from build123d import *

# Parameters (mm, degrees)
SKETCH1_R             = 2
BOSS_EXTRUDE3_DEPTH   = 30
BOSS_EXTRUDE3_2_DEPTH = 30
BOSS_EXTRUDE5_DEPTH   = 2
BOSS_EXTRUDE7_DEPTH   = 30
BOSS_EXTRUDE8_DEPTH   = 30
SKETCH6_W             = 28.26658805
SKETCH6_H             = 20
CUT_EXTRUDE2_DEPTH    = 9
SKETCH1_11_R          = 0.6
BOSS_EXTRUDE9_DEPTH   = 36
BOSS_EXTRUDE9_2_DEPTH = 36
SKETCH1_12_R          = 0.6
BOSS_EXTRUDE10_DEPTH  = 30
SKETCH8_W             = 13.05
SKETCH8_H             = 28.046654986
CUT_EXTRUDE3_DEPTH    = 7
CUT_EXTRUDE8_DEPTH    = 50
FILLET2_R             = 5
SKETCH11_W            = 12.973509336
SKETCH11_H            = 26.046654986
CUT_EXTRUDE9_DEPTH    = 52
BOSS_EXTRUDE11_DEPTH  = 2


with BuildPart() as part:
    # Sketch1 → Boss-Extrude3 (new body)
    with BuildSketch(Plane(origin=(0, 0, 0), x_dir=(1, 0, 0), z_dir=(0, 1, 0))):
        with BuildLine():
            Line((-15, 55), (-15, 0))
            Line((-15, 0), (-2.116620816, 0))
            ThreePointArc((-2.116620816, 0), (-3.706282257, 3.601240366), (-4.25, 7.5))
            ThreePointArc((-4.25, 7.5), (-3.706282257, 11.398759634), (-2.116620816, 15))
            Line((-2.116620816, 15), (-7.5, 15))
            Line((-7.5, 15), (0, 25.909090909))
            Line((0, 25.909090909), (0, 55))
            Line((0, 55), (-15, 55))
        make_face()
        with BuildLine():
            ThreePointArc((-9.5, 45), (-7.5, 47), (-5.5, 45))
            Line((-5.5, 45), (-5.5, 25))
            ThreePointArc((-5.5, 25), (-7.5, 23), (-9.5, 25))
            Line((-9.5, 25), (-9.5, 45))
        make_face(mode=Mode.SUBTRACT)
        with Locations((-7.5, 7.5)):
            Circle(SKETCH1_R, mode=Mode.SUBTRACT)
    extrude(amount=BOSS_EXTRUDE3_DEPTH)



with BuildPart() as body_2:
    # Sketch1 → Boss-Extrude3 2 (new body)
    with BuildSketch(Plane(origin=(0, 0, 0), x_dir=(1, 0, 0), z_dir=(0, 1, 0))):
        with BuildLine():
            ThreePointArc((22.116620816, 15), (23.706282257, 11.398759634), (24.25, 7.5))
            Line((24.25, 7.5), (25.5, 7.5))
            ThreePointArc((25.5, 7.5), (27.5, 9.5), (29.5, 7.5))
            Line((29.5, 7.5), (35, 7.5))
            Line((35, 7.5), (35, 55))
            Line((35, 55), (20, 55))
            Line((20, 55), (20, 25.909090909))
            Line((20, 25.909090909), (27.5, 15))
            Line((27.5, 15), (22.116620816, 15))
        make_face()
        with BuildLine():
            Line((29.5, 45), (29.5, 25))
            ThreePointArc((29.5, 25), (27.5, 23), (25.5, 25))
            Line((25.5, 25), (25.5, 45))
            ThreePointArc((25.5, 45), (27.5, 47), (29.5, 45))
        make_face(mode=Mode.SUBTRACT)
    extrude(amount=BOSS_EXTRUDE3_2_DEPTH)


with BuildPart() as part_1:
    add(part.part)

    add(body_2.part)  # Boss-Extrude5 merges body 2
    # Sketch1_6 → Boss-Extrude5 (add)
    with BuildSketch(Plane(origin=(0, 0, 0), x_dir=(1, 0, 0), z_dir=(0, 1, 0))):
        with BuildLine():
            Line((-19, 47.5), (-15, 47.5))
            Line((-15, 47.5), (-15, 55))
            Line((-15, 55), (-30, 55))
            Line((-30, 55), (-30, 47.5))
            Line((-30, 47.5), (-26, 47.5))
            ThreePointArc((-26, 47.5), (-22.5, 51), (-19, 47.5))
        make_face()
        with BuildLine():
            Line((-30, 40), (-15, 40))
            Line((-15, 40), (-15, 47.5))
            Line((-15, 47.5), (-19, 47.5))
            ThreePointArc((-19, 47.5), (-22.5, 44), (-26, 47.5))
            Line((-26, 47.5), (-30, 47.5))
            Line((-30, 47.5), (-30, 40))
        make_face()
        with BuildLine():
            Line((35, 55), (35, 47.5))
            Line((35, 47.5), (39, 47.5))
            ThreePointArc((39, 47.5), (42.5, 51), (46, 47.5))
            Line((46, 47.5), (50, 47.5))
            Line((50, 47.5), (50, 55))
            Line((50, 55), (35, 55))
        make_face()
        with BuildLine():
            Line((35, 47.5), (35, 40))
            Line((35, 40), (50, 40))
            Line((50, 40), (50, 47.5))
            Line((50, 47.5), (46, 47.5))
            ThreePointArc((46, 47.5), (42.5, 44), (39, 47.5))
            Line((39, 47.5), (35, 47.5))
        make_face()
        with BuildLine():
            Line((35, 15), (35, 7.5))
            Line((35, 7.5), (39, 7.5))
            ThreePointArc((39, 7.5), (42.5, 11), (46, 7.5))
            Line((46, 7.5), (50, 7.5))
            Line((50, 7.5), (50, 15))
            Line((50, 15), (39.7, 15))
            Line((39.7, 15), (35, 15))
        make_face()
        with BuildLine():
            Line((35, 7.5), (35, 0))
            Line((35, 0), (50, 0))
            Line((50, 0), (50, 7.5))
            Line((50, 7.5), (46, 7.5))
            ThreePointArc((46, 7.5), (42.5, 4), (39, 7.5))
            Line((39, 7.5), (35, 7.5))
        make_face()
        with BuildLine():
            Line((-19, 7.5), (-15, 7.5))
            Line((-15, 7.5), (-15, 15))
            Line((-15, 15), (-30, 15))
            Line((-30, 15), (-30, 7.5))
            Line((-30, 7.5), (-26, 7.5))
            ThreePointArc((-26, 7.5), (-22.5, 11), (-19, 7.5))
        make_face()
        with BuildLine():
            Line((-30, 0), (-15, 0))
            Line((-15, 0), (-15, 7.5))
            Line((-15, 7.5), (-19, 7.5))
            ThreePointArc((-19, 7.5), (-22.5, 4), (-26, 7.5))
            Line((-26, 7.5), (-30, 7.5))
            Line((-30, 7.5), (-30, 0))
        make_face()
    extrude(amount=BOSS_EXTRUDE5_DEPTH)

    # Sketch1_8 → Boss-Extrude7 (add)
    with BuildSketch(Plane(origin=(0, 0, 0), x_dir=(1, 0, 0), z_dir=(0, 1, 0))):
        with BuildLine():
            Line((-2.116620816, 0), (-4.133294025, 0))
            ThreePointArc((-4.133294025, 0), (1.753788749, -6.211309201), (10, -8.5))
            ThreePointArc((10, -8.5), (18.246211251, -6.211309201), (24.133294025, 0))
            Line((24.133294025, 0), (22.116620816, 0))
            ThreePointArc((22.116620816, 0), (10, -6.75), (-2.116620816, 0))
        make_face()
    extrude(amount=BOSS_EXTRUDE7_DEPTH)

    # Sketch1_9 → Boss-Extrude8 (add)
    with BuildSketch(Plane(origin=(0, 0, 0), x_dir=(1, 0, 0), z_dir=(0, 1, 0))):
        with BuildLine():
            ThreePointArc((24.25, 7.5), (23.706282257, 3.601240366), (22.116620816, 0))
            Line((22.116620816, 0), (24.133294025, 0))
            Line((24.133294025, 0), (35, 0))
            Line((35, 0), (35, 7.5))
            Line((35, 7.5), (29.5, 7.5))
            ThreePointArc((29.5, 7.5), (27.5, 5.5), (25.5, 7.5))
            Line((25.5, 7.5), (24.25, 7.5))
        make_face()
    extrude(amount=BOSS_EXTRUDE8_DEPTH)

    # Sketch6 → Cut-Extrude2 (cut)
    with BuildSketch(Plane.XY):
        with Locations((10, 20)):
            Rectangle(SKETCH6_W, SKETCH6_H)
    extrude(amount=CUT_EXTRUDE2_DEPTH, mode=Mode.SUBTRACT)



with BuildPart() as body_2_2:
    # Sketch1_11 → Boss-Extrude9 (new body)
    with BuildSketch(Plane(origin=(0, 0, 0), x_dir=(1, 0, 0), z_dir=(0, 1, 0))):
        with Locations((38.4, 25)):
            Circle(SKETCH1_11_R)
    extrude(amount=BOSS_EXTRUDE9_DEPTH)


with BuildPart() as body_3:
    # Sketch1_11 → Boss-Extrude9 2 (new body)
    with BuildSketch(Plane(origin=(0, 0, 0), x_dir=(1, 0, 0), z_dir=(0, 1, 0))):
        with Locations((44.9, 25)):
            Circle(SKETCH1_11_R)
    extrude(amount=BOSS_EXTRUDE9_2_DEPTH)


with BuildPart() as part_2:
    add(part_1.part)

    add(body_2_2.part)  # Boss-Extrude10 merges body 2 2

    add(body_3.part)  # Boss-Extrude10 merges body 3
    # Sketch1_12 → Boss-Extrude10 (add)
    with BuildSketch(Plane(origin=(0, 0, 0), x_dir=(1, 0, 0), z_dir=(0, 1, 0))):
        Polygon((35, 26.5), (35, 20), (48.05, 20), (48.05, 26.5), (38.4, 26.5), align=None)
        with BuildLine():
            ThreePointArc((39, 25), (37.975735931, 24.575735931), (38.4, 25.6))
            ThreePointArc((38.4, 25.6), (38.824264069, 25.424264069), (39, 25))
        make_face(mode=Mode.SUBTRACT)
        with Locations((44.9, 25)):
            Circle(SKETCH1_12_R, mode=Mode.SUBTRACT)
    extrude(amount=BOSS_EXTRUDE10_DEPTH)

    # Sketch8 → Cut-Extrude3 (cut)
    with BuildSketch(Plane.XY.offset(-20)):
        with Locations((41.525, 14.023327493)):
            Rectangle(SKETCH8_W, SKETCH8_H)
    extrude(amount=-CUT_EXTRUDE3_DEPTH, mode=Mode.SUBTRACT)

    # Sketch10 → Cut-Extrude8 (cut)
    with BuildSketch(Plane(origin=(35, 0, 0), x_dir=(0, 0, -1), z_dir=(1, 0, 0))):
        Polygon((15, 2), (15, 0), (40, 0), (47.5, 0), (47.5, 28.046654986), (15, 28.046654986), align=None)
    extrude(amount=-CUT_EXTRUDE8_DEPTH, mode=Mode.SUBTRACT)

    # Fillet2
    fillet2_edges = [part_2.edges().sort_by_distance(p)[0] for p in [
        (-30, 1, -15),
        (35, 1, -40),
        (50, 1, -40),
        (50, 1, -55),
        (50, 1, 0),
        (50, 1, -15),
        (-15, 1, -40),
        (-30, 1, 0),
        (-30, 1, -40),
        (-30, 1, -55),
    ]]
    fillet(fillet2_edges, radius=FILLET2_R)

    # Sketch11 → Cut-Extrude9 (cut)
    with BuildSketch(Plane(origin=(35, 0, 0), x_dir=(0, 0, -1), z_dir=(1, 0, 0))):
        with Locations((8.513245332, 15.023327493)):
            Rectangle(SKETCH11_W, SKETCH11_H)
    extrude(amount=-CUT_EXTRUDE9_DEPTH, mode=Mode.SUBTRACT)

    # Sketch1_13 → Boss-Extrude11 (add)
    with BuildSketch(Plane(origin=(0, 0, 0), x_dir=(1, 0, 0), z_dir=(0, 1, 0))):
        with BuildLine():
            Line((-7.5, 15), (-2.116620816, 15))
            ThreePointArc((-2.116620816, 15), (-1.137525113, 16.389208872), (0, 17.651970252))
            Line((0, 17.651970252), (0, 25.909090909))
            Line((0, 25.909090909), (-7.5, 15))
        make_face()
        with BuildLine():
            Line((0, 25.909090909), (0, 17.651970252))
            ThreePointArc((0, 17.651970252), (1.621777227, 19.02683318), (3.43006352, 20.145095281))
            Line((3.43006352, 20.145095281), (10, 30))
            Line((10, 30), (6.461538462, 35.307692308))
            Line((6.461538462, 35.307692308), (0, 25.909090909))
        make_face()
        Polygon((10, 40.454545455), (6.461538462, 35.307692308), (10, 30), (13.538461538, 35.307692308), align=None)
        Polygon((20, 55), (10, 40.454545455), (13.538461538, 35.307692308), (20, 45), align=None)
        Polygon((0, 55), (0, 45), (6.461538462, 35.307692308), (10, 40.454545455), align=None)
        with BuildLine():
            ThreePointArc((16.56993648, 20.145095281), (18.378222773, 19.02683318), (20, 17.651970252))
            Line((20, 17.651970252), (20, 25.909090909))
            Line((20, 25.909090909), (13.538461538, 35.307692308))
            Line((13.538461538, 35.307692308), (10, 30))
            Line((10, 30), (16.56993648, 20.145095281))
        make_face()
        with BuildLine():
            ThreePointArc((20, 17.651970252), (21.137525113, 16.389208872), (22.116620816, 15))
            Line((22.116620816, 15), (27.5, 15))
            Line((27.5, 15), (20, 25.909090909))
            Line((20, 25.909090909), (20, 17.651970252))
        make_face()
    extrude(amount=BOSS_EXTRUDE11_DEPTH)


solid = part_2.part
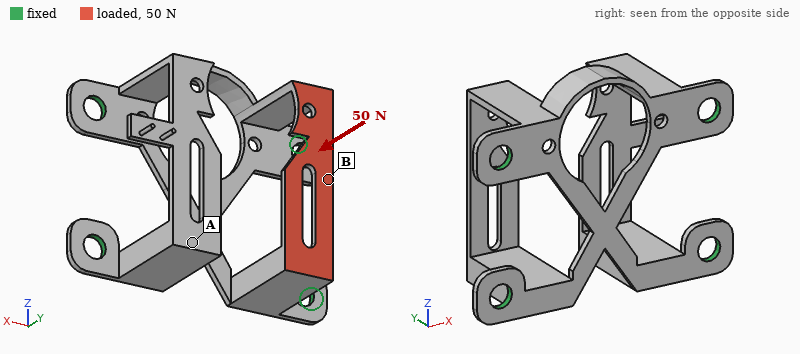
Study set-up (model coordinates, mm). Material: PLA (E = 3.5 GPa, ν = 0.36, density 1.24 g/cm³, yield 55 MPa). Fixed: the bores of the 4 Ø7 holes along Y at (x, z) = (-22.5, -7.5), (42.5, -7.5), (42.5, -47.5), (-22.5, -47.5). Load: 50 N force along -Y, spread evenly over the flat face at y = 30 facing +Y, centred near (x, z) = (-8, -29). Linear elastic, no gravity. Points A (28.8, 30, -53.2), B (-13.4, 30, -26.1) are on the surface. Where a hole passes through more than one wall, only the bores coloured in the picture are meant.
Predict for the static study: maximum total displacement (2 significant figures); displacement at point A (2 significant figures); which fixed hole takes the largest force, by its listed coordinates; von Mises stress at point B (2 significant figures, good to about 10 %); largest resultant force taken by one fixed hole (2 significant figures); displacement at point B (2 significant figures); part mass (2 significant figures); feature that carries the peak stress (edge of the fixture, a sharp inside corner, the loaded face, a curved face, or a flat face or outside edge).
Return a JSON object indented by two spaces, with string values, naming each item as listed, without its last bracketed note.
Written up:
{
  "maximum total displacement": "1.1 mm",
  "displacement at point A": "0.36 mm",
  "which fixed hole takes the largest force, by its listed coordinates": "(-22.5, -47.5)",
  "von Mises stress at point B": "15 MPa",
  "largest resultant force taken by one fixed hole": "29 N",
  "displacement at point B": "0.90 mm",
  "part mass": "17 g",
  "feature that carries the peak stress": "the loaded face"
}
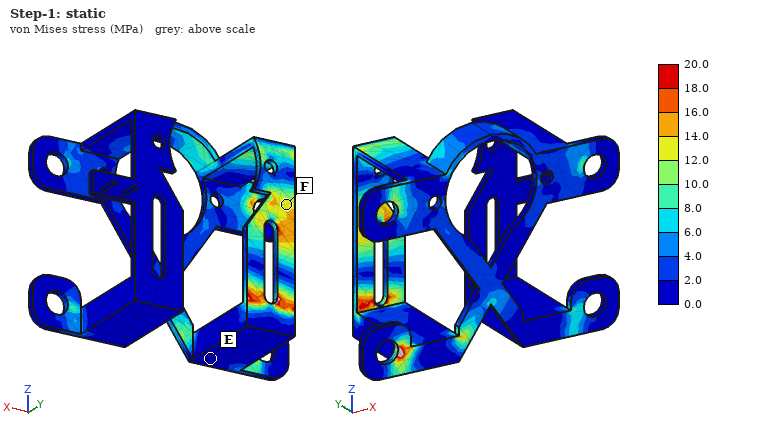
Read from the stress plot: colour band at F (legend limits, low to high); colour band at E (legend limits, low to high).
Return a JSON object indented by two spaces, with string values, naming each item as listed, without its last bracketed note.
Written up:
{
  "colour band at F": "12.0 to 14.0 MPa",
  "colour band at E": "0.0 to 2.0 MPa"
}
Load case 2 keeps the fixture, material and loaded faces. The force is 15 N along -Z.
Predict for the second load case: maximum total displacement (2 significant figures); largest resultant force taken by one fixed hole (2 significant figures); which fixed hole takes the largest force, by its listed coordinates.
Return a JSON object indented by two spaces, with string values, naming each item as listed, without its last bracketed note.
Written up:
{
  "maximum total displacement": "0.76 mm",
  "largest resultant force taken by one fixed hole": "10 N",
  "which fixed hole takes the largest force, by its listed coordinates": "(-22.5, -47.5)"
}
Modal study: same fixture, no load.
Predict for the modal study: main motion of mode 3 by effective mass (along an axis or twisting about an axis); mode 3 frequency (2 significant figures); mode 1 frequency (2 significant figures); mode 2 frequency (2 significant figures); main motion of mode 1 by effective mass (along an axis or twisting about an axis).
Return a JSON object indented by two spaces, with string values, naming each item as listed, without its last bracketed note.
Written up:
{
  "main motion of mode 3 by effective mass": "along Z",
  "mode 3 frequency": "410 Hz",
  "mode 1 frequency": "310 Hz",
  "mode 2 frequency": "390 Hz",
  "main motion of mode 1 by effective mass": "along Y"
}
